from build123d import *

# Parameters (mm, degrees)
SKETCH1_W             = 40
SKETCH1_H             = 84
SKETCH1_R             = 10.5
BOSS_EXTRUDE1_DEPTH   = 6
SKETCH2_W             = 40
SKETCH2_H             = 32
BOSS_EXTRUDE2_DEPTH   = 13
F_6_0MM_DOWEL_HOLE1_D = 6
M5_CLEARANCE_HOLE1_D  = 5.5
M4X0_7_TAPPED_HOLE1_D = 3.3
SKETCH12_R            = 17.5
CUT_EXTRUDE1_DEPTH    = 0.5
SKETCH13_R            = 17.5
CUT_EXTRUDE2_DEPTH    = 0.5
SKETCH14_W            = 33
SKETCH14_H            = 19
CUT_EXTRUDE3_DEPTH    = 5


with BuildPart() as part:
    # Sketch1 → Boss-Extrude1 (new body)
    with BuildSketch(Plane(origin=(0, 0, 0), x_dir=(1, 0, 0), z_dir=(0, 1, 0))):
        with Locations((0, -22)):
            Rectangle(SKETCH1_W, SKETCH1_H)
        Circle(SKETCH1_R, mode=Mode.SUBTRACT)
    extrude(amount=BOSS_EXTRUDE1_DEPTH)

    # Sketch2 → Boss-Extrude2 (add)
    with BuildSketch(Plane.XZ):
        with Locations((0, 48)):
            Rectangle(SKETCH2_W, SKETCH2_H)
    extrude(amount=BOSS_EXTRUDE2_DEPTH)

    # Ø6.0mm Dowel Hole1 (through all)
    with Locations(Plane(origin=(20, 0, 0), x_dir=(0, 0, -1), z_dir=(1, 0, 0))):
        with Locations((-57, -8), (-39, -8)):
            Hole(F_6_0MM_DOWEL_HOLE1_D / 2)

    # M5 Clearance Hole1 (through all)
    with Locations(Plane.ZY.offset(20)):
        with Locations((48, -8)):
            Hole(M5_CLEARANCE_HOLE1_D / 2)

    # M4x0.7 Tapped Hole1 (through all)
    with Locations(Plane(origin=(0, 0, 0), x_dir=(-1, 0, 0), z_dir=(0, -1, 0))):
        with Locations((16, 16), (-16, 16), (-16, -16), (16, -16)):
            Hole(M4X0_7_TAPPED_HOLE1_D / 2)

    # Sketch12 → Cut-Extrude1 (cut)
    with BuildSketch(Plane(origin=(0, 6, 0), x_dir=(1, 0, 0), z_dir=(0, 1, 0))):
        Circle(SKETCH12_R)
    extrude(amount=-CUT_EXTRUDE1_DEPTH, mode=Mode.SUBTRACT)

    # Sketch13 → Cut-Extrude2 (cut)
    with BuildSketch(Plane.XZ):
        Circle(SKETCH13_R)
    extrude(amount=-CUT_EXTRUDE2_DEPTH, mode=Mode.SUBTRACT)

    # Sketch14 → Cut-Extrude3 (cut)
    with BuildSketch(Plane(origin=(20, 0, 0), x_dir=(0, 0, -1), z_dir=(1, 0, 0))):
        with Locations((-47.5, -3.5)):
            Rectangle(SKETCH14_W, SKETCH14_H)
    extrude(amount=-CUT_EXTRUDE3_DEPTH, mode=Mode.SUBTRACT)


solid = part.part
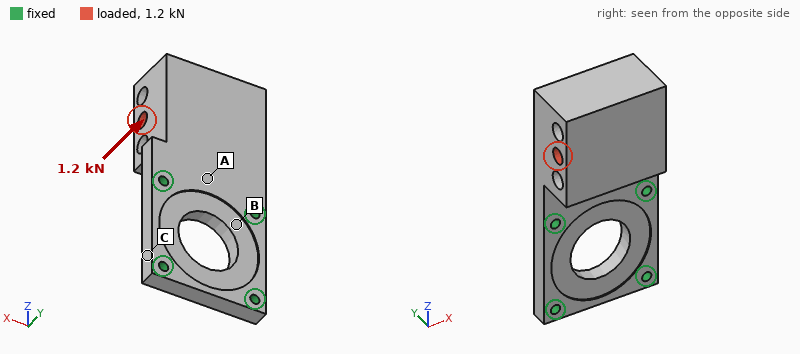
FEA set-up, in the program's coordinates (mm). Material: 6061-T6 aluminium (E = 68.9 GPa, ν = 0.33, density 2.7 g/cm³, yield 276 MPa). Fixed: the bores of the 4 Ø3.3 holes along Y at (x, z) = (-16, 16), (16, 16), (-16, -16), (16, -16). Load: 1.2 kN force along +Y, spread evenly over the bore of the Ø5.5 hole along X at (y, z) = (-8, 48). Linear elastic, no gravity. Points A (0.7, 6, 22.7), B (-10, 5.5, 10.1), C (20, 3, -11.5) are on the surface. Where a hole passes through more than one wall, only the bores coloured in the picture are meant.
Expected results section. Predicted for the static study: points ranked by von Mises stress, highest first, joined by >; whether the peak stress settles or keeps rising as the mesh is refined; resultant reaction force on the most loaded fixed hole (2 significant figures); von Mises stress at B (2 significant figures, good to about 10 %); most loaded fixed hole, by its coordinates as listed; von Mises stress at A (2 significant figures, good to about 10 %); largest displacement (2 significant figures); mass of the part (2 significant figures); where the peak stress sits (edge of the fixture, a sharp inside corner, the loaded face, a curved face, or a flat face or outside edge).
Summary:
A > B > C
keeps rising
800 N
56 MPa
(-16, 16)
81 MPa
0.57 mm
76 g
edge of the fixture
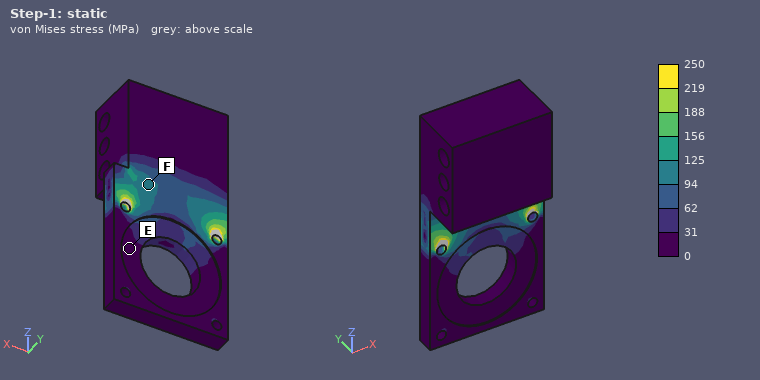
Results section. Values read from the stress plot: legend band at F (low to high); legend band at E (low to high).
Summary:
94 to 125 MPa
0 to 31 MPa
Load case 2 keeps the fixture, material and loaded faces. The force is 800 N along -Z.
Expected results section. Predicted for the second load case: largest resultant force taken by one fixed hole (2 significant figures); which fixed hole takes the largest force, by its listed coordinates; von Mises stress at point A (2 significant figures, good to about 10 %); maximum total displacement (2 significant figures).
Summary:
440 N
(-16, 16)
24 MPa
0.17 mm
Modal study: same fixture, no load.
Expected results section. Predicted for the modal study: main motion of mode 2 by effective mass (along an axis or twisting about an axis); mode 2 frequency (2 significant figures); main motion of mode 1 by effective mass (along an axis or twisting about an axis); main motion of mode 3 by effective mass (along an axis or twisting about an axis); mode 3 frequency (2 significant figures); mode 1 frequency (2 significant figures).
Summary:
along X
5000 Hz
along Y
along X
7100 Hz
1200 Hz
